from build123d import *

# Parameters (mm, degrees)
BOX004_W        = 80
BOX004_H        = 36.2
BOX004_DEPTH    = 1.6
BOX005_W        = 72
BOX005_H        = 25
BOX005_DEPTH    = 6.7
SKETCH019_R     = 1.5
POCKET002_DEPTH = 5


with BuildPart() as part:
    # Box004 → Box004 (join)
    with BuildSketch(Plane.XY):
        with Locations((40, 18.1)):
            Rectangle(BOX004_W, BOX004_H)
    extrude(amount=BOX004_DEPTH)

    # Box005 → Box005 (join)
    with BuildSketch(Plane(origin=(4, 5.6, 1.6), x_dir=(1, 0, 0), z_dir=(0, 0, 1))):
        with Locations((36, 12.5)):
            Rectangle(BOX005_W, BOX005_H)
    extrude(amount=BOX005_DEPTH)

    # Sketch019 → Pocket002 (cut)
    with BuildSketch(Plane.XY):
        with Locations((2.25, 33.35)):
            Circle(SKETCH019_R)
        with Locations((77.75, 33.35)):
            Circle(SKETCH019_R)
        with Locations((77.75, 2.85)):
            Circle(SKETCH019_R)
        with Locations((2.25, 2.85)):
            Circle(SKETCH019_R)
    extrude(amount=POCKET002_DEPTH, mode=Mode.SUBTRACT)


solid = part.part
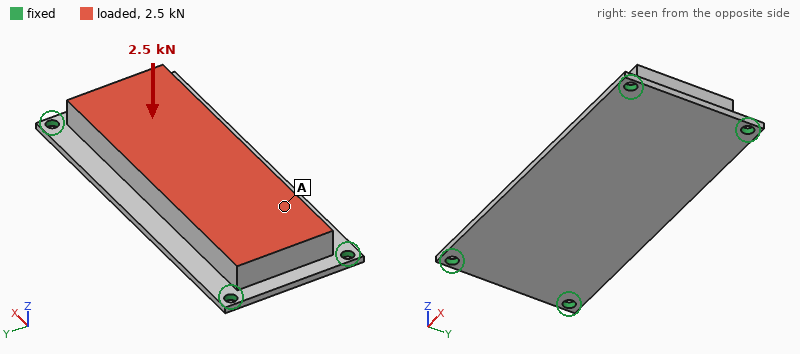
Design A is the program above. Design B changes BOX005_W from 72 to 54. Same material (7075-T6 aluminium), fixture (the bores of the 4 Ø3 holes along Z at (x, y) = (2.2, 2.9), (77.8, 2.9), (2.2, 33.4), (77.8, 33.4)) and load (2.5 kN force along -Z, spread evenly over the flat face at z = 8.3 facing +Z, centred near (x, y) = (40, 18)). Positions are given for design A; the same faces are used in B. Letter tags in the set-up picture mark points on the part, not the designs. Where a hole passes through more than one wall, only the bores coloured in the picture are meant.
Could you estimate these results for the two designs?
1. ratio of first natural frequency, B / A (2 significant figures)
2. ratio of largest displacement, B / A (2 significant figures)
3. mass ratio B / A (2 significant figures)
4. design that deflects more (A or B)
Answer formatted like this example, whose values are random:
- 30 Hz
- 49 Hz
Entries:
- 0.57
- 3.2
- 0.82
- B
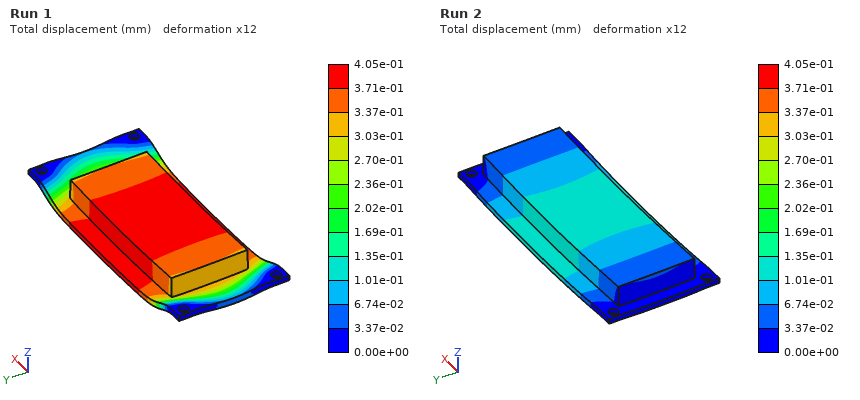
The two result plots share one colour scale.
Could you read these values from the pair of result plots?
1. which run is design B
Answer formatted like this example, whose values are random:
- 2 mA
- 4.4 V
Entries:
- Run 1
